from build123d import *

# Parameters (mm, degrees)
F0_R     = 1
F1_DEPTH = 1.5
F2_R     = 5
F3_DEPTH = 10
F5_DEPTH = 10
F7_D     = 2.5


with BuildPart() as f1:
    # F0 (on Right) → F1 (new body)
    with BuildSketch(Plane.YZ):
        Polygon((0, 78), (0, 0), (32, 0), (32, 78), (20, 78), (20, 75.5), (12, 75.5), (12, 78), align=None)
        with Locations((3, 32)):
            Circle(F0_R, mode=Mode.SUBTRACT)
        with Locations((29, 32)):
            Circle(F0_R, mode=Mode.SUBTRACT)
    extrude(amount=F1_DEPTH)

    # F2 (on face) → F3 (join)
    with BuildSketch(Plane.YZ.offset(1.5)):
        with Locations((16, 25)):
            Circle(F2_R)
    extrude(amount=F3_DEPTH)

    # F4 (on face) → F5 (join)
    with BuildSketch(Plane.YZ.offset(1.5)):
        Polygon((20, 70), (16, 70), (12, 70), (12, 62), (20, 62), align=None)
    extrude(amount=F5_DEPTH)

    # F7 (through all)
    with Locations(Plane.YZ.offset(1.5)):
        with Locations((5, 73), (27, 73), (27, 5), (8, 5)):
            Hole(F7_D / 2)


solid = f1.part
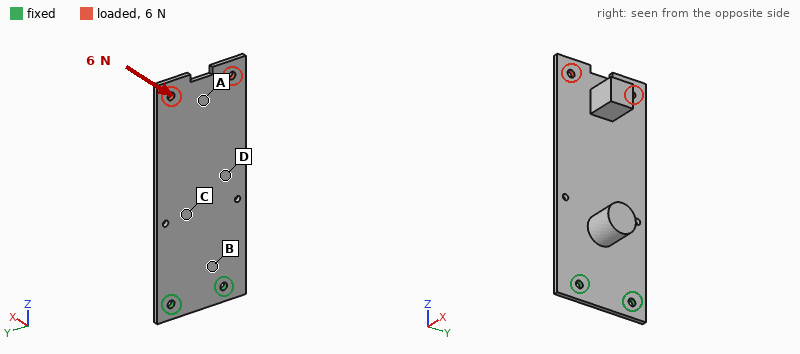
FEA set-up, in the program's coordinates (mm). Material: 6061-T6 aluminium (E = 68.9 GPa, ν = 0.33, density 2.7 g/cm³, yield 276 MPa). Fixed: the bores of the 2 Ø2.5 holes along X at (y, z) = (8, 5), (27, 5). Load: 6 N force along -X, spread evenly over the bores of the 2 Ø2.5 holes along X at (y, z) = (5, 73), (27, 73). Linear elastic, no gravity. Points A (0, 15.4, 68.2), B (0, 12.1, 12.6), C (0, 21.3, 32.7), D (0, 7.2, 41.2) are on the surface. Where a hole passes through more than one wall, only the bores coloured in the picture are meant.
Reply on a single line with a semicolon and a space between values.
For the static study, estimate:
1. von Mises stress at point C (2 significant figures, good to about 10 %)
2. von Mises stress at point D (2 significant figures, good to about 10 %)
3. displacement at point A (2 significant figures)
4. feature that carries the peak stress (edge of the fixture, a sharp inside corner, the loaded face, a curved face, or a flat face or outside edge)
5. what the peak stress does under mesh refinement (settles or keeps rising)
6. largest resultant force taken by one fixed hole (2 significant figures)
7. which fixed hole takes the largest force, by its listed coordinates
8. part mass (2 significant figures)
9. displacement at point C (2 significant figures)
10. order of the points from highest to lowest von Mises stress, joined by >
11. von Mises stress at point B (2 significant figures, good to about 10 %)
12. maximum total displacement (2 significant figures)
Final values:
22 MPa; 15 MPa; 0.79 mm; edge of the fixture; keeps rising; 4.0 N; (8, 5); 14 g; 0.20 mm; B > C > D > A; 27 MPa; 0.99 mm
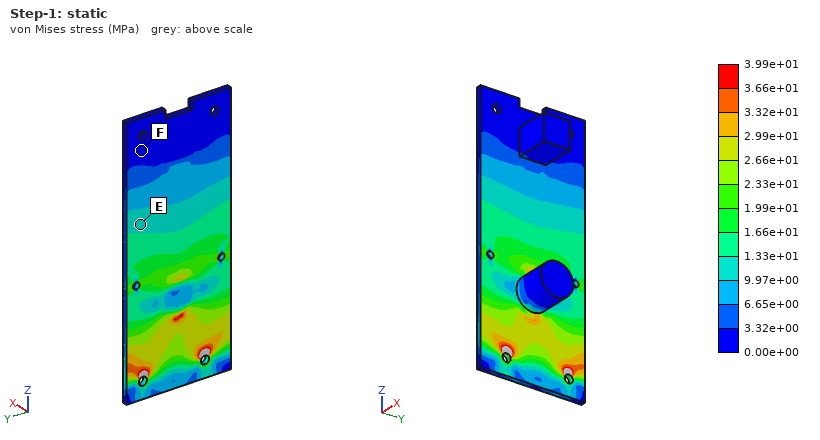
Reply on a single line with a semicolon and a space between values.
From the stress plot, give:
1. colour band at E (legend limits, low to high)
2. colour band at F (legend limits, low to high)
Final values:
9.97e+00 to 1.33e+01 MPa; 0.00e+00 to 3.32e+00 MPa
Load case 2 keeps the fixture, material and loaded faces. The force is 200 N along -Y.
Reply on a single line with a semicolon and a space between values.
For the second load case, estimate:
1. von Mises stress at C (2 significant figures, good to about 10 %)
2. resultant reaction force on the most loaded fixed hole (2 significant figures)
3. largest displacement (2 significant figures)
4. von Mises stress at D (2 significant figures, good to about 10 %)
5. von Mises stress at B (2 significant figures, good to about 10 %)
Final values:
15 MPa; 680 N; 0.12 mm; 16 MPa; 25 MPa
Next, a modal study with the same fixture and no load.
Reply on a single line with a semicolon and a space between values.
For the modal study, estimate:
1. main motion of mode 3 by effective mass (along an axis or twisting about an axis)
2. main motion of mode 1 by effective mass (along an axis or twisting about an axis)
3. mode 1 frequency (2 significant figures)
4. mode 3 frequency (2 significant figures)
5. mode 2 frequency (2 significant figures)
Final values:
along X; along X; 210 Hz; 1300 Hz; 1100 Hz
